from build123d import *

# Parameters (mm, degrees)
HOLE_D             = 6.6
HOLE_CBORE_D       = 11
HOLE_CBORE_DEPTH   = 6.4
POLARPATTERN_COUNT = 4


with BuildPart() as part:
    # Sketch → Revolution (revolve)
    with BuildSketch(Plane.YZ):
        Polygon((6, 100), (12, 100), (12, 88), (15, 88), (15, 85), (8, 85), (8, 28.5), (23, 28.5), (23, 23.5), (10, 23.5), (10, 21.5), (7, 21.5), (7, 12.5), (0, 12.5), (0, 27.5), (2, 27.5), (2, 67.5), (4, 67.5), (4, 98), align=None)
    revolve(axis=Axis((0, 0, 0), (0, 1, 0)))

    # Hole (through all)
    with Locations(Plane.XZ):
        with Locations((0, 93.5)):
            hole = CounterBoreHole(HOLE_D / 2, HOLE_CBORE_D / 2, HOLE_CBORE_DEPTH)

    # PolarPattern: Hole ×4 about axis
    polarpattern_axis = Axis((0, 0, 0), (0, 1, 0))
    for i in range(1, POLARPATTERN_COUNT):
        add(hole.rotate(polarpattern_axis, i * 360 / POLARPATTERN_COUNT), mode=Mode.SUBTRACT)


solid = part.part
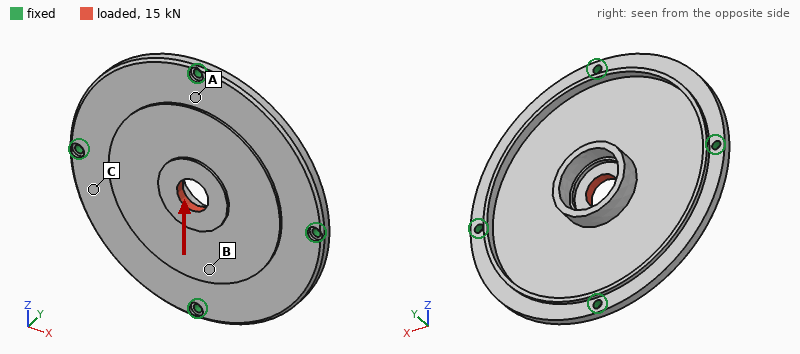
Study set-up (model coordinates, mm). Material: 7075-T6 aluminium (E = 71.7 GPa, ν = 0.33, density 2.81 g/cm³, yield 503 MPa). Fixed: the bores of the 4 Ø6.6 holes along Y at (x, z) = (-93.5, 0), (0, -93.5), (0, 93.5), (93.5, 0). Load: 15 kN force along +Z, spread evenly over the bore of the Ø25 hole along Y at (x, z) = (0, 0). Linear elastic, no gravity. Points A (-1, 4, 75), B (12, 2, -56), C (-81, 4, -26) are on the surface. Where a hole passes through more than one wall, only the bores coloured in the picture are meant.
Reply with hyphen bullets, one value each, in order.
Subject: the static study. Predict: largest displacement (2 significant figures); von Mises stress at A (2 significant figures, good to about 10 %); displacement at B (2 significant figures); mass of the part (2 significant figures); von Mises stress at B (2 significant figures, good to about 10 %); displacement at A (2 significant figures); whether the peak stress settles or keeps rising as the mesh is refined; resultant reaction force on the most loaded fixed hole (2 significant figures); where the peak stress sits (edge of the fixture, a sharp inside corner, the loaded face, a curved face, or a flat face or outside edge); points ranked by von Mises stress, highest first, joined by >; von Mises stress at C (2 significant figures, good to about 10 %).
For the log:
- 34 µm
- 33 MPa
- 19 µm
- 570 g
- 17 MPa
- 15 µm
- keeps rising
- 4.3 kN
- edge of the fixture
- A > B > C
- 7.0 MPa
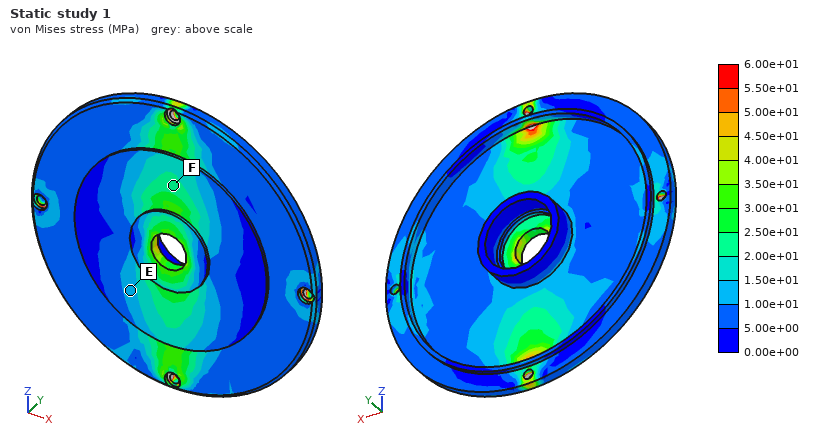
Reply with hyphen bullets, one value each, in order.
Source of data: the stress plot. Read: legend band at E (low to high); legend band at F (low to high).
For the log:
- 1.00e+01 to 1.50e+01 MPa
- 2.00e+01 to 2.50e+01 MPa
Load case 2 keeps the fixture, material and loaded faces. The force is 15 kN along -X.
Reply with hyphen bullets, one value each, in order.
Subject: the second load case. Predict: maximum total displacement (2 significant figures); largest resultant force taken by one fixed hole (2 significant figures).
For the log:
- 34 µm
- 4.3 kN
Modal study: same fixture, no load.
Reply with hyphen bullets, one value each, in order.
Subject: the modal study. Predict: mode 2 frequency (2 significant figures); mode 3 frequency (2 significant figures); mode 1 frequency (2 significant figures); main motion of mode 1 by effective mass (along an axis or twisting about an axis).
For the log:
- 1800 Hz
- 1800 Hz
- 1300 Hz
- along Y
